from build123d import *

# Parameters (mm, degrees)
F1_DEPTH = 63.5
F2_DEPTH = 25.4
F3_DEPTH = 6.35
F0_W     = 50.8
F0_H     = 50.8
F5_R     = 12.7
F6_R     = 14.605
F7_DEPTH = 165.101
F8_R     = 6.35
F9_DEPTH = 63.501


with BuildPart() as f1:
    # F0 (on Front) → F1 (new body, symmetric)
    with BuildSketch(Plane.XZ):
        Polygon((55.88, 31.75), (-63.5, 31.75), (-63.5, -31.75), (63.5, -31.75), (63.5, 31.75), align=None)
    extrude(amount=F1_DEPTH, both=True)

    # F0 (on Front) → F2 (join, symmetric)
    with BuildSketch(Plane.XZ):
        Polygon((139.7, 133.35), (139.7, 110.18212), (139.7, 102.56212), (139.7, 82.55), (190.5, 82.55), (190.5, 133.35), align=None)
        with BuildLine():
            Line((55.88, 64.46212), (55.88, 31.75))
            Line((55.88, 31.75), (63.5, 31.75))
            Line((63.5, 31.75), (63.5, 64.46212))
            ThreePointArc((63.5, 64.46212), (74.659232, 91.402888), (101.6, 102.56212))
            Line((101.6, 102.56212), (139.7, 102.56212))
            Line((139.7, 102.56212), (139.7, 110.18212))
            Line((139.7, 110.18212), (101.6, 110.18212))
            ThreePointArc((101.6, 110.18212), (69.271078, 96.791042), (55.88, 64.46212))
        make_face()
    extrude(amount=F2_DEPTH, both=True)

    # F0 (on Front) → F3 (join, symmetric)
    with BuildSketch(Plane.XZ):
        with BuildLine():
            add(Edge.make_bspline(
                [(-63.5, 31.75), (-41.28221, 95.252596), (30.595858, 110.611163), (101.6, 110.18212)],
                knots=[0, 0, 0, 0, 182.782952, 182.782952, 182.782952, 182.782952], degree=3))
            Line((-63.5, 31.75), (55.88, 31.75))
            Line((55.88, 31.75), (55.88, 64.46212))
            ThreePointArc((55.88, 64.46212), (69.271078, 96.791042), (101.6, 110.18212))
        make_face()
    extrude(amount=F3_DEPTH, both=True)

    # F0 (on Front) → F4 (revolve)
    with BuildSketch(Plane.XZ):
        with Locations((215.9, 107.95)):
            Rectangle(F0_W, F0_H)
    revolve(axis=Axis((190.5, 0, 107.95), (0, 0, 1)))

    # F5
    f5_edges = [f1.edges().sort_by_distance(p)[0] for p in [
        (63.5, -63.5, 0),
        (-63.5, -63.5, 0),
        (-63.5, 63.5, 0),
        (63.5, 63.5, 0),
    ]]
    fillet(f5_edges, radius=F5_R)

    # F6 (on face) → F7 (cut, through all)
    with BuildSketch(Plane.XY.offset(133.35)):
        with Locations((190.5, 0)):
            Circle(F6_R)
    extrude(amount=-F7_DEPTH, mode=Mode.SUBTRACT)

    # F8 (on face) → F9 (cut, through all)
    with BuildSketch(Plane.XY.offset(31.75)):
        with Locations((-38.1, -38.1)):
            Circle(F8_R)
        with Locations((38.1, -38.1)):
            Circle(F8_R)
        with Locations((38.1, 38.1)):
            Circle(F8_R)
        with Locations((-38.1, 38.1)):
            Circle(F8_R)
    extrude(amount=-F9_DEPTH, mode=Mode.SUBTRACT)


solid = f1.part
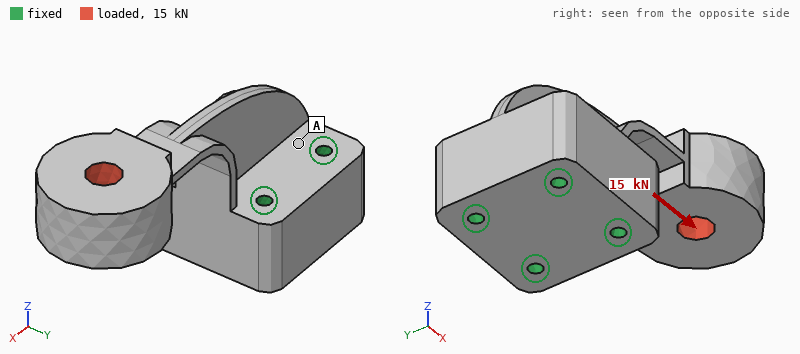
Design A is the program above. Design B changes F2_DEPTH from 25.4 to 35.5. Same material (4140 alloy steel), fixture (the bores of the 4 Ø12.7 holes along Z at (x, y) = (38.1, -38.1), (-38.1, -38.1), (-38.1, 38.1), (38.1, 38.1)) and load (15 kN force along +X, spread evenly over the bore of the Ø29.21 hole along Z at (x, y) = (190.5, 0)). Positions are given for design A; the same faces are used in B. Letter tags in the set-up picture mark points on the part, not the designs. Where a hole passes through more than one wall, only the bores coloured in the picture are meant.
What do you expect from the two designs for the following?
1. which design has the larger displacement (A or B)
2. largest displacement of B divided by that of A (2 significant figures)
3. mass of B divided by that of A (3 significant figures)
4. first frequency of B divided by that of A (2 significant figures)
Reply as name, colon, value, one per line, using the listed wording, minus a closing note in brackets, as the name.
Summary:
which design has the larger displacement: A
largest displacement of B divided by that of A: 0.81
mass of B divided by that of A: 1.02
first frequency of B divided by that of A: 1.2
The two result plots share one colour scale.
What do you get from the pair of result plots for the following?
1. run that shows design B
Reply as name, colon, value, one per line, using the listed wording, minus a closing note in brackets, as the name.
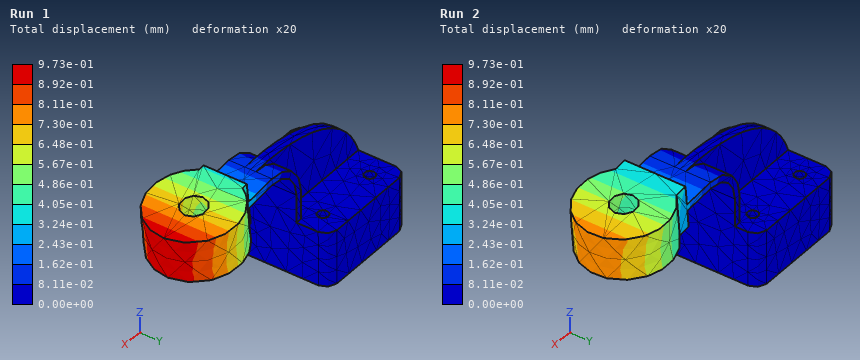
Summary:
run that shows design B: Run 2
